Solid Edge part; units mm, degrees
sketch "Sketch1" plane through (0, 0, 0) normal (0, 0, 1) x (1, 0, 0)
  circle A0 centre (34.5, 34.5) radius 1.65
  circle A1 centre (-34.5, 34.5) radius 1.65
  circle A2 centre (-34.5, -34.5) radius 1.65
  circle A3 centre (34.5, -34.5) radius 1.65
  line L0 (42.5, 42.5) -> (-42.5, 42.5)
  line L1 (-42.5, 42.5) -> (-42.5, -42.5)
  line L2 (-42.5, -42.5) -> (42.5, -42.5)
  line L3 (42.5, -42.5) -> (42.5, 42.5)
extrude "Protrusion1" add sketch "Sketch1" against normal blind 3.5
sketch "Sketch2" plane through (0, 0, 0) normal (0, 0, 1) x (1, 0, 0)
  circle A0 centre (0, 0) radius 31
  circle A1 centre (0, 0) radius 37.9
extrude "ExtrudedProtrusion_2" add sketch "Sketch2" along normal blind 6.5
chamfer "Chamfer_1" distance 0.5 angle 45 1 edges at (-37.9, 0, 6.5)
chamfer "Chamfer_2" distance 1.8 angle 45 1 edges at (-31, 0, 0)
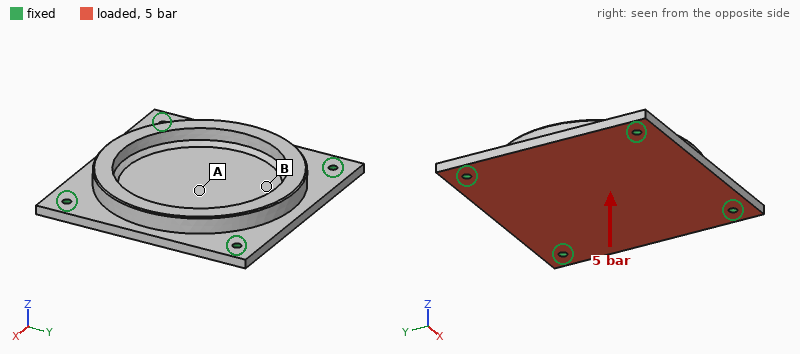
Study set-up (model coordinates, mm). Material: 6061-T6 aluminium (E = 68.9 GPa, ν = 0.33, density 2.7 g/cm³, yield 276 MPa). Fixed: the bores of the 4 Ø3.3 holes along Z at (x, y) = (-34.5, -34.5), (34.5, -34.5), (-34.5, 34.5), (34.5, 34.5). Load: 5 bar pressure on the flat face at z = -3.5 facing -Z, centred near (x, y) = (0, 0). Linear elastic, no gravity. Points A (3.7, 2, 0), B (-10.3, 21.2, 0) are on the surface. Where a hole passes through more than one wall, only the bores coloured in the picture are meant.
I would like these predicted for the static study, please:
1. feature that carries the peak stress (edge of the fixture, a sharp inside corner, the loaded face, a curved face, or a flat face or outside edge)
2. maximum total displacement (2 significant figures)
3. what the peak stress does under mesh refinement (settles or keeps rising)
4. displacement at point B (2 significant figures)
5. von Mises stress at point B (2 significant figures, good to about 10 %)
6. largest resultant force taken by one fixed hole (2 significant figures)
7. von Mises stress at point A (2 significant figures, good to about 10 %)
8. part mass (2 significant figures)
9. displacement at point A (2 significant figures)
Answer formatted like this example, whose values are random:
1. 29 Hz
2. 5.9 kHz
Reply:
1. edge of the fixture
2. 0.13 mm
3. keeps rising
4. 0.087 mm
5. 12 MPa
6. 1.0 kN
7. 27 MPa
8. 95 g
9. 0.13 mm
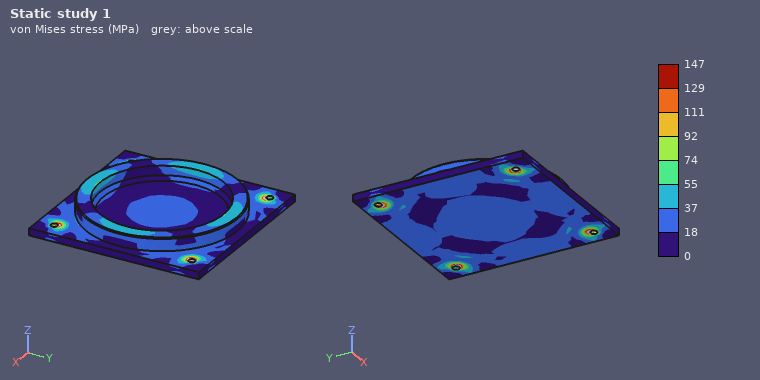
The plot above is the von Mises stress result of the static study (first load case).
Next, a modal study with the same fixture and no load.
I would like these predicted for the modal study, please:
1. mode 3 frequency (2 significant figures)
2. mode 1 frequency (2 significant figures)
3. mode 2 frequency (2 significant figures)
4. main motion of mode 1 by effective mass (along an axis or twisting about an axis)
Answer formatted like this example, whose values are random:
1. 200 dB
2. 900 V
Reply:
1. 5100 Hz
2. 3600 Hz
3. 5100 Hz
4. along Z
